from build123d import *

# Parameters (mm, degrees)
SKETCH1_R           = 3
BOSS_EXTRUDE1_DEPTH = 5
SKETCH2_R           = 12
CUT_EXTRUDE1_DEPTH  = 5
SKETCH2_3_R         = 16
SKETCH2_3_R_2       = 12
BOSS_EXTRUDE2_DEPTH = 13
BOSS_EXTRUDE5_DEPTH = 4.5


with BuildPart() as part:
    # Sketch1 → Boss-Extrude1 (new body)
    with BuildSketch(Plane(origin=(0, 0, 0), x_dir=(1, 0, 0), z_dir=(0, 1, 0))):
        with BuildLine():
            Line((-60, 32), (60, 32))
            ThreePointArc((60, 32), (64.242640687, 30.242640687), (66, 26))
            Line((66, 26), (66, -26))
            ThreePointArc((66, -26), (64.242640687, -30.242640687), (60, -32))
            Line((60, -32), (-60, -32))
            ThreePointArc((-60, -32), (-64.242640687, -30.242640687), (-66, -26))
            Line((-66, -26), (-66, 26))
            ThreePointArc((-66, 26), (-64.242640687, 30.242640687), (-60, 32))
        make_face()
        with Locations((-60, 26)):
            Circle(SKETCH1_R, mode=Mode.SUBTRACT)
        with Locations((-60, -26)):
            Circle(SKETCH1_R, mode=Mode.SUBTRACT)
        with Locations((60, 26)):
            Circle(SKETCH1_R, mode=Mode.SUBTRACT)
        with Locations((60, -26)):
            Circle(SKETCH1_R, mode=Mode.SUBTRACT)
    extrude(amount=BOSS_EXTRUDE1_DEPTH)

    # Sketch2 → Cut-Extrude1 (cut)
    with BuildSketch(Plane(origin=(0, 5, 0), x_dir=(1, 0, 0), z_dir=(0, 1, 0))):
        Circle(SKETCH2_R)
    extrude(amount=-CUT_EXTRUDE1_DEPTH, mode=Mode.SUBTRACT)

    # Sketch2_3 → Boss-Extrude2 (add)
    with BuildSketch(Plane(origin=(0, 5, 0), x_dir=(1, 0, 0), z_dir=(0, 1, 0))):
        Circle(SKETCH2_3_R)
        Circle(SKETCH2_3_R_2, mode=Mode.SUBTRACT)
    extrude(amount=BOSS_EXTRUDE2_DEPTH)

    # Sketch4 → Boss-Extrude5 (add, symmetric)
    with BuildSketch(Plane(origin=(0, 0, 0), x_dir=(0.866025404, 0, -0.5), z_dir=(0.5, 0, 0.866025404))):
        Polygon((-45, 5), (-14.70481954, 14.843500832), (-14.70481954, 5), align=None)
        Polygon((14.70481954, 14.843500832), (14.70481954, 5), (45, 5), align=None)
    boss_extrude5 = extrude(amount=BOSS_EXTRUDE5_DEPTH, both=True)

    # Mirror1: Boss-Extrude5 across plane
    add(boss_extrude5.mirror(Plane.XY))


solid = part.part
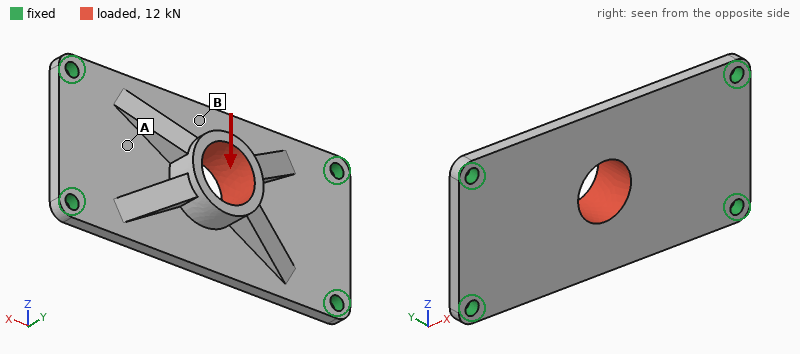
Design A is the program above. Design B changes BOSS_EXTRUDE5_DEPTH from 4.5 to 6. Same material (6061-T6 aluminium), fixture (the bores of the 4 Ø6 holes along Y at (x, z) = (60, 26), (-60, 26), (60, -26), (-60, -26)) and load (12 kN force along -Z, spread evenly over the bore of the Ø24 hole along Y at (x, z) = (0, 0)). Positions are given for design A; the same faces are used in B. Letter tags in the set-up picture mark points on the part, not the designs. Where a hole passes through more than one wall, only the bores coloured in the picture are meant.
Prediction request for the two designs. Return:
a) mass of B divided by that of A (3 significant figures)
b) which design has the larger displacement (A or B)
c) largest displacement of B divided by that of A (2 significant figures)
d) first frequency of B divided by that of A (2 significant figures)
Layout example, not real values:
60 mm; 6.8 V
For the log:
1.04; A; 0.88; 1.0
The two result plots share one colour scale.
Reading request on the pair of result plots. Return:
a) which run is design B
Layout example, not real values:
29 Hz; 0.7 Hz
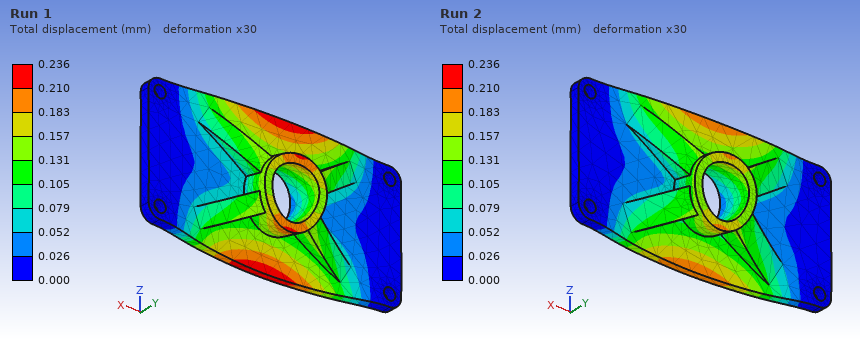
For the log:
Run 2
